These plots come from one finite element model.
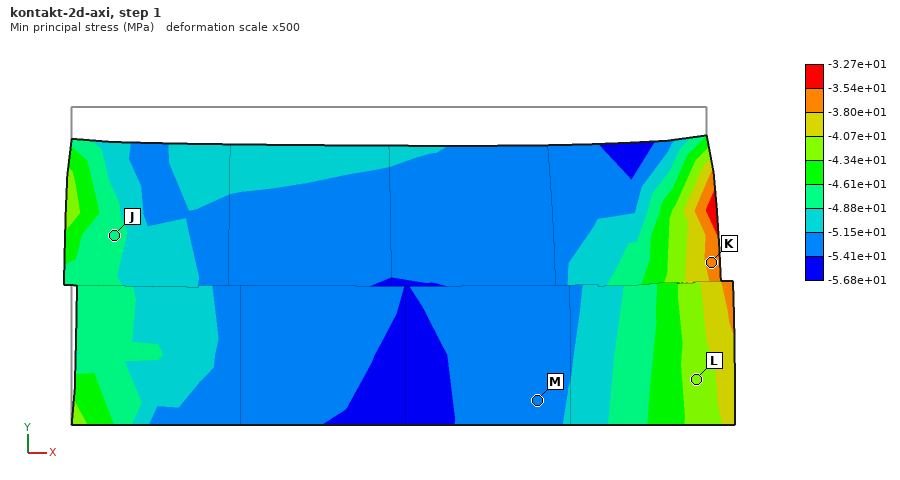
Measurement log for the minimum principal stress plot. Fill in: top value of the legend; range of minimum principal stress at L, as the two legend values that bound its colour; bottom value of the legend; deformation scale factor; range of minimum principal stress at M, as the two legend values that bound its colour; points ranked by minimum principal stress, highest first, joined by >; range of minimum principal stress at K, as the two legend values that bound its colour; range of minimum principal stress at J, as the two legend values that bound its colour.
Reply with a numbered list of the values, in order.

1. -3.27e+01 MPa
2. -4.34e+01 to -4.07e+01 MPa
3. -5.68e+01 MPa
4. 500
5. -5.41e+01 to -5.15e+01 MPa
6. K > L > J > M
7. -3.80e+01 to -3.54e+01 MPa
8. -4.88e+01 to -4.61e+01 MPa
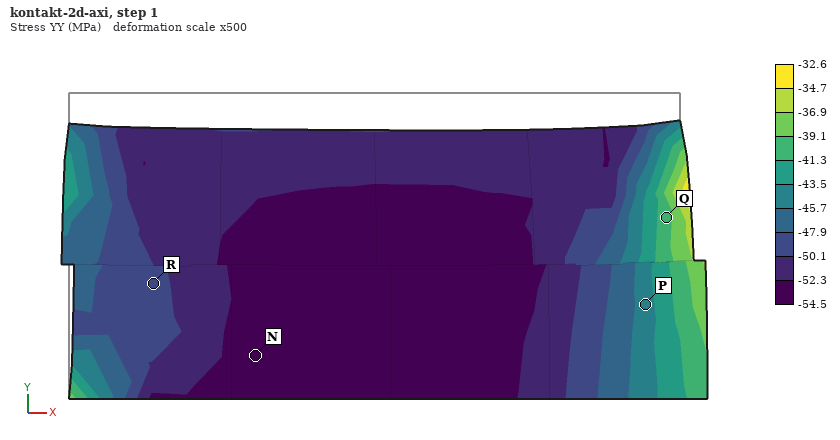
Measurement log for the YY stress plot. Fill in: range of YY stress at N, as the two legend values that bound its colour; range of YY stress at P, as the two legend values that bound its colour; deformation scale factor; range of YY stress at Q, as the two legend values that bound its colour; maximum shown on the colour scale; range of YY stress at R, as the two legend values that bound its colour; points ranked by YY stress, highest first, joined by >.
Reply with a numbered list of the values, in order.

1. -54.5 to -52.3 MPa
2. -45.7 to -43.5 MPa
3. 500
4. -41.3 to -39.1 MPa
5. -32.6 MPa
6. -50.1 to -47.9 MPa
7. Q > P > R > N
